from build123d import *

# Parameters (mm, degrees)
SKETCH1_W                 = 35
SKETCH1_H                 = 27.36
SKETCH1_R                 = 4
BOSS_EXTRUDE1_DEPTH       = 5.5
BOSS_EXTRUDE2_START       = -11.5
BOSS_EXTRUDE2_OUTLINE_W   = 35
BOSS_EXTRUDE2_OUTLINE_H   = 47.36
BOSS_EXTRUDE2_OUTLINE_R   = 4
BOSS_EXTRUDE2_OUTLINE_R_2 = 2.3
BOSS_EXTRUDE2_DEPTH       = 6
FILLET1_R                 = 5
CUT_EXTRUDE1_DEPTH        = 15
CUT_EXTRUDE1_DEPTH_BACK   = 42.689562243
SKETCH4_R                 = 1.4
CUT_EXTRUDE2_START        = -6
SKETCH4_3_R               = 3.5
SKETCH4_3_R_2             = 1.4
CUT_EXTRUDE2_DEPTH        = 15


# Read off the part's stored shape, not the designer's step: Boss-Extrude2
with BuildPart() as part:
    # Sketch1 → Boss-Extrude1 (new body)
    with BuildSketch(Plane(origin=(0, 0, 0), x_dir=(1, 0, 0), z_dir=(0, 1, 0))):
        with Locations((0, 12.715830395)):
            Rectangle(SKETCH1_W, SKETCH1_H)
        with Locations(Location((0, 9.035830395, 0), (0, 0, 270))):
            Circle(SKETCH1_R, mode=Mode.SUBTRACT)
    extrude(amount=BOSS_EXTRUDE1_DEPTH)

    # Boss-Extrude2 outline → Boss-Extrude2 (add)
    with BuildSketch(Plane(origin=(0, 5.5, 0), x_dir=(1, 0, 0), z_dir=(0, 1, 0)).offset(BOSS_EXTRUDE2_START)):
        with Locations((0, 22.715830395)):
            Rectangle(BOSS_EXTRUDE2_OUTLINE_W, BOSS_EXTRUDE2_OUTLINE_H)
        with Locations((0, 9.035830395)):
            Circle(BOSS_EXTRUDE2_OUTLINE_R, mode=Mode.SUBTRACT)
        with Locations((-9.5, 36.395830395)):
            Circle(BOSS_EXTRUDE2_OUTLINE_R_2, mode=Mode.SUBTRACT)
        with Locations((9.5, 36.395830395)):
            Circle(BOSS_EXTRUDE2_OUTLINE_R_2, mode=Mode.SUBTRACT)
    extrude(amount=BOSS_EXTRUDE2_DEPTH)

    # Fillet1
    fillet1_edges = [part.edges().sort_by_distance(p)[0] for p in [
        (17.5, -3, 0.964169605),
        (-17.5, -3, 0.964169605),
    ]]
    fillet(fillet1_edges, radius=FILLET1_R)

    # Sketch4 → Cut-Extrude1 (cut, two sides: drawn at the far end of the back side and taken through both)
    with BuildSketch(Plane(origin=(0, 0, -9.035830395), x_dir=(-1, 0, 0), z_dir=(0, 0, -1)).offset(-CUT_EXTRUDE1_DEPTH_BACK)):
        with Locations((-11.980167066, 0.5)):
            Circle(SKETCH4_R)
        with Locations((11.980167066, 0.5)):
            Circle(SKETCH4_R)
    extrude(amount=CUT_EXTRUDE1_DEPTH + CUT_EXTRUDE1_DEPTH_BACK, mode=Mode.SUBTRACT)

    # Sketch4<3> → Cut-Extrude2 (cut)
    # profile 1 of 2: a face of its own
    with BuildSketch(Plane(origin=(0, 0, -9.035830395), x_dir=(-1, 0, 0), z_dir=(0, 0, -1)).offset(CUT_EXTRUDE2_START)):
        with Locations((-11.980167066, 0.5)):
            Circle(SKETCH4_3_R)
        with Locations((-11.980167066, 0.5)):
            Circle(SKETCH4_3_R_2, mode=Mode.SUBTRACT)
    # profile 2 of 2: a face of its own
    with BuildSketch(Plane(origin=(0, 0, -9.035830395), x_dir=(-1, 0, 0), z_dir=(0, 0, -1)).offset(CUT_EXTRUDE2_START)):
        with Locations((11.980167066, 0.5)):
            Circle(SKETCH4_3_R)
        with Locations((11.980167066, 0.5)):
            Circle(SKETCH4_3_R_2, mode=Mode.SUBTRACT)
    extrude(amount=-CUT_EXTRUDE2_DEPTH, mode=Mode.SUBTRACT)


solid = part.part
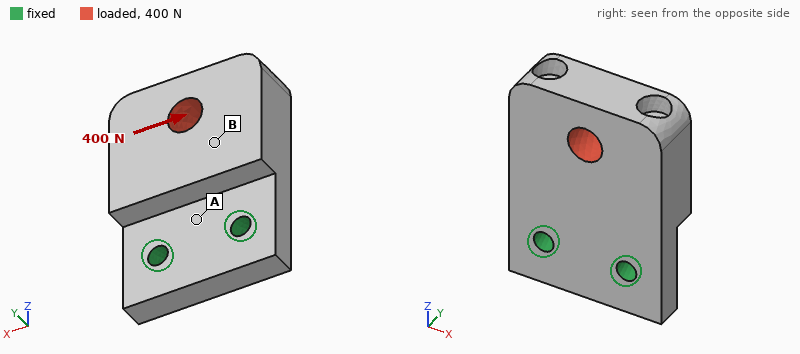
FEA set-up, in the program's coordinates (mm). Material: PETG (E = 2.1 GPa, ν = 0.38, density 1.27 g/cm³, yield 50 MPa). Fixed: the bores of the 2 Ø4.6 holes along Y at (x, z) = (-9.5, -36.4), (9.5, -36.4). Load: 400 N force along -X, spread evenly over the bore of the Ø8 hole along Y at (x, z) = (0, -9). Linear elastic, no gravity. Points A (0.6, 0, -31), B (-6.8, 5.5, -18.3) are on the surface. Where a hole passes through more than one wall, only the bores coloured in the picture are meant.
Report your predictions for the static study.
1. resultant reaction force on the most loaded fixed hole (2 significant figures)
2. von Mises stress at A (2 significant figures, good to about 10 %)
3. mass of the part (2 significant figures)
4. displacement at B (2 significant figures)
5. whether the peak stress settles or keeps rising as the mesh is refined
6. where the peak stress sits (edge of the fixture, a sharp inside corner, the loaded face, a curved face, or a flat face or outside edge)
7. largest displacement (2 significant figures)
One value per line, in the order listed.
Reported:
530 N
5.5 MPa
17 g
0.100 mm
keeps rising
edge of the fixture
0.20 mm
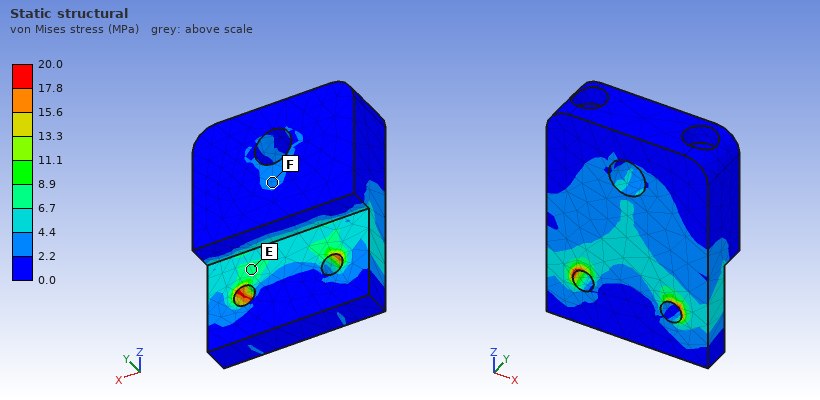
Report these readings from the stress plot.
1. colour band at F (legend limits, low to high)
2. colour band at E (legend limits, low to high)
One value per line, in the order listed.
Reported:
2.2 to 4.4 MPa
6.7 to 8.9 MPa
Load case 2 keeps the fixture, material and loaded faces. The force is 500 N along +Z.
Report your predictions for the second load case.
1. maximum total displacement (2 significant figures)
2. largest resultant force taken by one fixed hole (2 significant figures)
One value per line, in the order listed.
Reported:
0.40 mm
250 N
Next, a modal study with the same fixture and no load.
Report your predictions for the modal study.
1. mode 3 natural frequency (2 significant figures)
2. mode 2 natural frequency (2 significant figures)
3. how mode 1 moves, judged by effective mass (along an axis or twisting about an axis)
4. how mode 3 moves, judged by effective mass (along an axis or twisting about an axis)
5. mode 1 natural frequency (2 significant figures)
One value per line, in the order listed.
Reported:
2600 Hz
2400 Hz
along Y
along X
770 Hz
